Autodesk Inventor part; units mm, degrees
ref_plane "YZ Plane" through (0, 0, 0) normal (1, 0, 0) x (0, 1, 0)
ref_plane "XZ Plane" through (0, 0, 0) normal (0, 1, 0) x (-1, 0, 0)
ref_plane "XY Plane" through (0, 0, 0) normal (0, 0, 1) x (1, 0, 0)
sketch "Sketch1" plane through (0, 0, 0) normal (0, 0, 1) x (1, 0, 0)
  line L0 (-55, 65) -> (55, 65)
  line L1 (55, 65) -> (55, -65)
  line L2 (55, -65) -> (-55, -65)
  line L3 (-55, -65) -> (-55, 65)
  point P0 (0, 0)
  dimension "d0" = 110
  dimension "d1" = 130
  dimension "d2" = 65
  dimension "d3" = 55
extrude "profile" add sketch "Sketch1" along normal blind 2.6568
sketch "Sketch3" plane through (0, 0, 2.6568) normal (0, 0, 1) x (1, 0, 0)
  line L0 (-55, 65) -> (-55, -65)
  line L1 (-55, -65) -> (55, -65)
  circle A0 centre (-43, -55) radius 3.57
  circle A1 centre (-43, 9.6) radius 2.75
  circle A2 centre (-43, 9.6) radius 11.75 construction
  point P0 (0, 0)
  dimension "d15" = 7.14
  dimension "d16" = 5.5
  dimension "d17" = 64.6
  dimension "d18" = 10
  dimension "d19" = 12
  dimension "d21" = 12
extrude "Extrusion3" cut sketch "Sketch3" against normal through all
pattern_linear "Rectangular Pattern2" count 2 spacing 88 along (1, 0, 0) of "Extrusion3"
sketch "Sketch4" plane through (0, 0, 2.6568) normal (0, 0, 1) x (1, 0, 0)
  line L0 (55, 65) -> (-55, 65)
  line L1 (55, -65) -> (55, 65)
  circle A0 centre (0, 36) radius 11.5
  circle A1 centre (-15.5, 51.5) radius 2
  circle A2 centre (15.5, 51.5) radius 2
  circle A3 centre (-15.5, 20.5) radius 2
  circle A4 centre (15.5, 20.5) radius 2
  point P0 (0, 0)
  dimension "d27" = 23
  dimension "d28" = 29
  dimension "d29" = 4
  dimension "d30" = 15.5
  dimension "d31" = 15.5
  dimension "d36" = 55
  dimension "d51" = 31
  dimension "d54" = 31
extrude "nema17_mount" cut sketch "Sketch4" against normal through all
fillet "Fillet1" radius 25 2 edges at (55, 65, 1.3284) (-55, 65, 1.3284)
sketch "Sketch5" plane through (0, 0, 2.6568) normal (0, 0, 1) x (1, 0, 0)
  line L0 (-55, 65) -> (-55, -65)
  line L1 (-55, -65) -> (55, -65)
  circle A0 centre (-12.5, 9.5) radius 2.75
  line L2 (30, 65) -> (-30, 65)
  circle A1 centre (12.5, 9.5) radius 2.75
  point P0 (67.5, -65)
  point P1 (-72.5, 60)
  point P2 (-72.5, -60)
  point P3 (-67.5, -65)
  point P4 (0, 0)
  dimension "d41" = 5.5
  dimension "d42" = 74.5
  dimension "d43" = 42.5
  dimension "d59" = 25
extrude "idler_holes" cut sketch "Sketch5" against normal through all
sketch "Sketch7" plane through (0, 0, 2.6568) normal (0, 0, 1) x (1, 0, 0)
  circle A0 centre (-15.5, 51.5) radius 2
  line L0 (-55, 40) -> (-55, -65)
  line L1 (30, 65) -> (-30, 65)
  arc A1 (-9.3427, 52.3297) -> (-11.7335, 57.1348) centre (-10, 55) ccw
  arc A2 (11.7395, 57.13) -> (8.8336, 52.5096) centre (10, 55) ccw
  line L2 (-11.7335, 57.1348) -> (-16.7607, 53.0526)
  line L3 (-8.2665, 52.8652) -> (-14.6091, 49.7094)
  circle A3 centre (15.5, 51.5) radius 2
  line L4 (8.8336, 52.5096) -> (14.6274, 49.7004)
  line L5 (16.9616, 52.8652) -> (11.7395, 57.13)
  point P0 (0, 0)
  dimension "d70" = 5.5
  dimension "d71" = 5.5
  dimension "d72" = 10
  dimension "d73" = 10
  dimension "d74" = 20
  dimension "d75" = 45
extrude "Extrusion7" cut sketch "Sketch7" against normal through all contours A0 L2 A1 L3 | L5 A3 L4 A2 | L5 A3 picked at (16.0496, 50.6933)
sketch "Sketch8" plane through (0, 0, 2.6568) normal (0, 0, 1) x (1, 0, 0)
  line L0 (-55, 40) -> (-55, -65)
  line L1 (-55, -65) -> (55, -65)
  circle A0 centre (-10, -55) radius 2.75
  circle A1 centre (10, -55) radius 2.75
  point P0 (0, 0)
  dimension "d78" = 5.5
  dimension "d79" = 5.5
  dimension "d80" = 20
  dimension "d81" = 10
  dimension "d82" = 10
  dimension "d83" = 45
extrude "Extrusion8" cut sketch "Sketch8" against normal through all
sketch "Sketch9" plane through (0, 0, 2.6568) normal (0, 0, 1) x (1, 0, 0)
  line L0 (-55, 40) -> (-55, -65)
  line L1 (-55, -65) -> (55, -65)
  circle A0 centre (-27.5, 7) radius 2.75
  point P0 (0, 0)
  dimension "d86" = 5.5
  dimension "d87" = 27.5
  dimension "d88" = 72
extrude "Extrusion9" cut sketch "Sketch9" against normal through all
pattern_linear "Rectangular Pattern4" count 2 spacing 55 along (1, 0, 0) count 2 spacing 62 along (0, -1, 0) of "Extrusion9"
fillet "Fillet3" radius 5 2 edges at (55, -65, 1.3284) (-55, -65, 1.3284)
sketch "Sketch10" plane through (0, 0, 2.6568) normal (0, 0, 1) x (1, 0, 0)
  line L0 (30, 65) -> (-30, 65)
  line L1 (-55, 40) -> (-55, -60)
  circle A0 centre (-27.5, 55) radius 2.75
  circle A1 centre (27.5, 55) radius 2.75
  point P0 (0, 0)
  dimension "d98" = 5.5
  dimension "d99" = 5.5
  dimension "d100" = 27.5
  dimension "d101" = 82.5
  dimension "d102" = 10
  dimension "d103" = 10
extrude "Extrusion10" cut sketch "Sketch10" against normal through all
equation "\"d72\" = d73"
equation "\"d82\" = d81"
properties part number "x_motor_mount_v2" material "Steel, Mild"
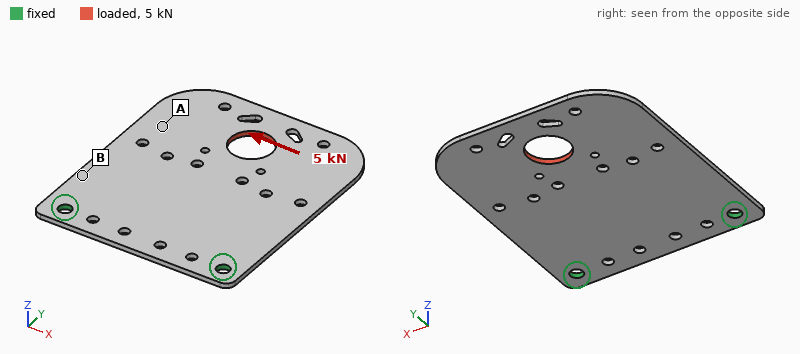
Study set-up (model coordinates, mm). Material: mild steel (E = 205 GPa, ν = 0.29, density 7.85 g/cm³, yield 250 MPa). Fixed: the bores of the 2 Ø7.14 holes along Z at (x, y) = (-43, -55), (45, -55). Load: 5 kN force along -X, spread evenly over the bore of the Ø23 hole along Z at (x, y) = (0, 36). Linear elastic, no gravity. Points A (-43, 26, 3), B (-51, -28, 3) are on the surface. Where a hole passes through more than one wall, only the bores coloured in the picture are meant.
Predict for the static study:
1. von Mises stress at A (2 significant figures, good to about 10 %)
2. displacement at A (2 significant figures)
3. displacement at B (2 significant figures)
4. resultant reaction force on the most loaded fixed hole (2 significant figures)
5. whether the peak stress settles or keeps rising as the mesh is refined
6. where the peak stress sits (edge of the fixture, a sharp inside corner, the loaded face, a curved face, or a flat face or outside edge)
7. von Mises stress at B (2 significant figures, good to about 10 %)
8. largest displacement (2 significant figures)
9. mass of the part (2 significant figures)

19 MPa
47 µm
18 µm
5.6 kN
keeps rising
edge of the fixture
55 MPa
66 µm
270 g
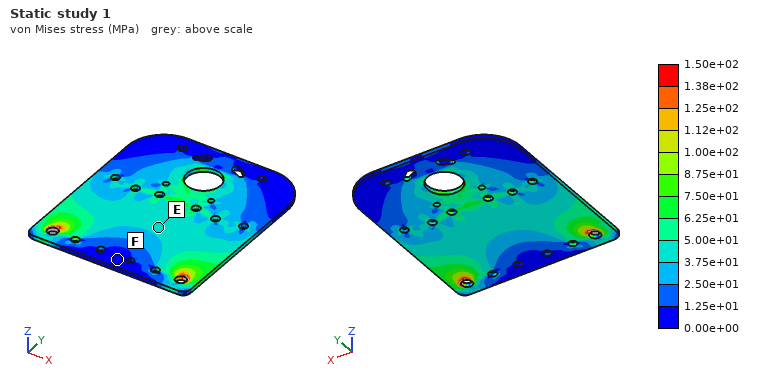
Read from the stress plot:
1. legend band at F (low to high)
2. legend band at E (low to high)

0.00e+00 to 1.25e+01 MPa
3.75e+01 to 5.00e+01 MPa
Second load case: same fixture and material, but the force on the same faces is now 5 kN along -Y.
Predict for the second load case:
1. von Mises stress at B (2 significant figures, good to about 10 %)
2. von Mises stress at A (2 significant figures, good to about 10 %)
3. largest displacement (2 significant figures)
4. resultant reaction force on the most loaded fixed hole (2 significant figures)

25 MPa
9.1 MPa
19 µm
2.6 kN
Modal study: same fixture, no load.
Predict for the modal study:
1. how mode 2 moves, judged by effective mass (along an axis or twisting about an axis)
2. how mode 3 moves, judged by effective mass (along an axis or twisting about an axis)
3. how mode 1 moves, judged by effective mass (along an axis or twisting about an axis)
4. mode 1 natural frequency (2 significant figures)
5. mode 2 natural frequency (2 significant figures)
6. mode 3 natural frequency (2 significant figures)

twisting about Y
along Z
along Z
150 Hz
430 Hz
890 Hz
